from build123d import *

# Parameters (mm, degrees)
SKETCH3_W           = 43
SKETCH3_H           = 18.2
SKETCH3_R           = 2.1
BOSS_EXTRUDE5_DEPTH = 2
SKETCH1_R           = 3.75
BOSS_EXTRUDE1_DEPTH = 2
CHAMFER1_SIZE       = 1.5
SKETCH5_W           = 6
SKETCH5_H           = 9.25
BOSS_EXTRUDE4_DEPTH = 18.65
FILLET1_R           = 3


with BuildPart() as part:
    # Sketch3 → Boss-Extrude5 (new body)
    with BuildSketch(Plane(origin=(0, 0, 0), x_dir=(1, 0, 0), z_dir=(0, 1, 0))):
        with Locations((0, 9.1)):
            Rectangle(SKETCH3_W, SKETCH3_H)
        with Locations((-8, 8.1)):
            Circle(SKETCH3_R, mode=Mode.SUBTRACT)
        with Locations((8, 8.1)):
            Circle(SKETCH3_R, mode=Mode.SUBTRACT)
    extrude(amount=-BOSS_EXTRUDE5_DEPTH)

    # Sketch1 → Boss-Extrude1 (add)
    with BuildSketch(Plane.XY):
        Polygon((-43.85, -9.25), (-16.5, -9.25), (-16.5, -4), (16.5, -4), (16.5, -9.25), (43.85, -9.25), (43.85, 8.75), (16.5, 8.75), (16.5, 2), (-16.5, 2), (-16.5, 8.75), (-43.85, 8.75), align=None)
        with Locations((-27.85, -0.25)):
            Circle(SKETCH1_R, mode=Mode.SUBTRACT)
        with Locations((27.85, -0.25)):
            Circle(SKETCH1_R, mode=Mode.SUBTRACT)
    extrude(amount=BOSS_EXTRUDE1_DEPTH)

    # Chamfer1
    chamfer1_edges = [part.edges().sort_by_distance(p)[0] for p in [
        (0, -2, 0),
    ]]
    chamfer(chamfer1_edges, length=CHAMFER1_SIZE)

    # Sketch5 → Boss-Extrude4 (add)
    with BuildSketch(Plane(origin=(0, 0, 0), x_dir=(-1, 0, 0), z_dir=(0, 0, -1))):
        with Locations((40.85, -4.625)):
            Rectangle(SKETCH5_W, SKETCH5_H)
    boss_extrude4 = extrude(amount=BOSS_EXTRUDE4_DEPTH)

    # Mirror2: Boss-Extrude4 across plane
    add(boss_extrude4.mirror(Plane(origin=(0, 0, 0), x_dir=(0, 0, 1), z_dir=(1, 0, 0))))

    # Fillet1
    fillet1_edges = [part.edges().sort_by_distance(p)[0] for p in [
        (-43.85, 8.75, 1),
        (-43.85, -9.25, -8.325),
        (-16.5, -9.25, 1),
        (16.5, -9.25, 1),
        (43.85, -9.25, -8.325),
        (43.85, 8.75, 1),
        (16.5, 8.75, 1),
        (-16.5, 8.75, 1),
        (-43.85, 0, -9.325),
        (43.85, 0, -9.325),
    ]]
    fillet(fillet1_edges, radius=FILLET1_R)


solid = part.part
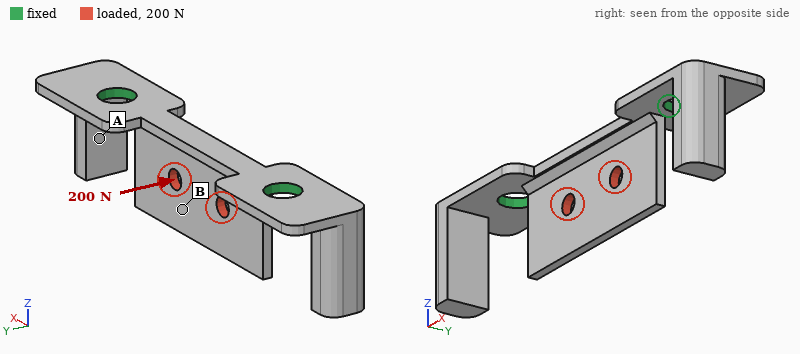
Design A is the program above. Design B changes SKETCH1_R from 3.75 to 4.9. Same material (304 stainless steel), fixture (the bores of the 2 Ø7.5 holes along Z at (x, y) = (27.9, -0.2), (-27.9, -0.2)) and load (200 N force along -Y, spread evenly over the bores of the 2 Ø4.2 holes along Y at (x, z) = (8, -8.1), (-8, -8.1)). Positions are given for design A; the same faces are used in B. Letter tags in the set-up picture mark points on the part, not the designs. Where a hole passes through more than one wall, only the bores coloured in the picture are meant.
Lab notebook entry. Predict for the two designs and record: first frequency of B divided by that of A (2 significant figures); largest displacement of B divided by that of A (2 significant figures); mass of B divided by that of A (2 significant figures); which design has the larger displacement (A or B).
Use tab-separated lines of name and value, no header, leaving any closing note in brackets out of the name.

first frequency of B divided by that of A	1.1
largest displacement of B divided by that of A	0.89
mass of B divided by that of A	0.98
which design has the larger displacement	A
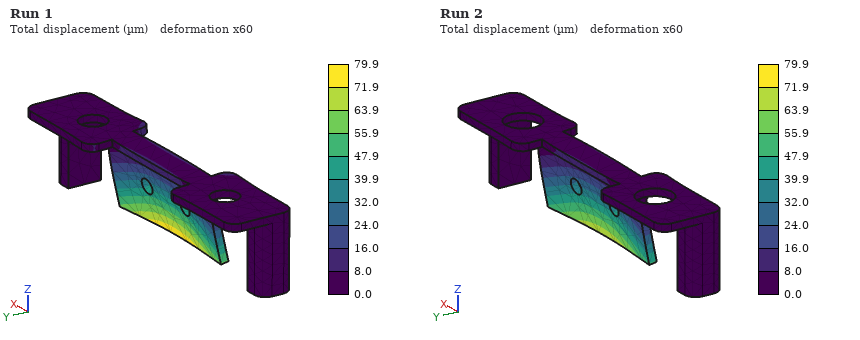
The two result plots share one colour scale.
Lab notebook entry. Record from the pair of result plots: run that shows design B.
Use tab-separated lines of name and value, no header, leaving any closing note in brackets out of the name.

run that shows design B	Run 2
